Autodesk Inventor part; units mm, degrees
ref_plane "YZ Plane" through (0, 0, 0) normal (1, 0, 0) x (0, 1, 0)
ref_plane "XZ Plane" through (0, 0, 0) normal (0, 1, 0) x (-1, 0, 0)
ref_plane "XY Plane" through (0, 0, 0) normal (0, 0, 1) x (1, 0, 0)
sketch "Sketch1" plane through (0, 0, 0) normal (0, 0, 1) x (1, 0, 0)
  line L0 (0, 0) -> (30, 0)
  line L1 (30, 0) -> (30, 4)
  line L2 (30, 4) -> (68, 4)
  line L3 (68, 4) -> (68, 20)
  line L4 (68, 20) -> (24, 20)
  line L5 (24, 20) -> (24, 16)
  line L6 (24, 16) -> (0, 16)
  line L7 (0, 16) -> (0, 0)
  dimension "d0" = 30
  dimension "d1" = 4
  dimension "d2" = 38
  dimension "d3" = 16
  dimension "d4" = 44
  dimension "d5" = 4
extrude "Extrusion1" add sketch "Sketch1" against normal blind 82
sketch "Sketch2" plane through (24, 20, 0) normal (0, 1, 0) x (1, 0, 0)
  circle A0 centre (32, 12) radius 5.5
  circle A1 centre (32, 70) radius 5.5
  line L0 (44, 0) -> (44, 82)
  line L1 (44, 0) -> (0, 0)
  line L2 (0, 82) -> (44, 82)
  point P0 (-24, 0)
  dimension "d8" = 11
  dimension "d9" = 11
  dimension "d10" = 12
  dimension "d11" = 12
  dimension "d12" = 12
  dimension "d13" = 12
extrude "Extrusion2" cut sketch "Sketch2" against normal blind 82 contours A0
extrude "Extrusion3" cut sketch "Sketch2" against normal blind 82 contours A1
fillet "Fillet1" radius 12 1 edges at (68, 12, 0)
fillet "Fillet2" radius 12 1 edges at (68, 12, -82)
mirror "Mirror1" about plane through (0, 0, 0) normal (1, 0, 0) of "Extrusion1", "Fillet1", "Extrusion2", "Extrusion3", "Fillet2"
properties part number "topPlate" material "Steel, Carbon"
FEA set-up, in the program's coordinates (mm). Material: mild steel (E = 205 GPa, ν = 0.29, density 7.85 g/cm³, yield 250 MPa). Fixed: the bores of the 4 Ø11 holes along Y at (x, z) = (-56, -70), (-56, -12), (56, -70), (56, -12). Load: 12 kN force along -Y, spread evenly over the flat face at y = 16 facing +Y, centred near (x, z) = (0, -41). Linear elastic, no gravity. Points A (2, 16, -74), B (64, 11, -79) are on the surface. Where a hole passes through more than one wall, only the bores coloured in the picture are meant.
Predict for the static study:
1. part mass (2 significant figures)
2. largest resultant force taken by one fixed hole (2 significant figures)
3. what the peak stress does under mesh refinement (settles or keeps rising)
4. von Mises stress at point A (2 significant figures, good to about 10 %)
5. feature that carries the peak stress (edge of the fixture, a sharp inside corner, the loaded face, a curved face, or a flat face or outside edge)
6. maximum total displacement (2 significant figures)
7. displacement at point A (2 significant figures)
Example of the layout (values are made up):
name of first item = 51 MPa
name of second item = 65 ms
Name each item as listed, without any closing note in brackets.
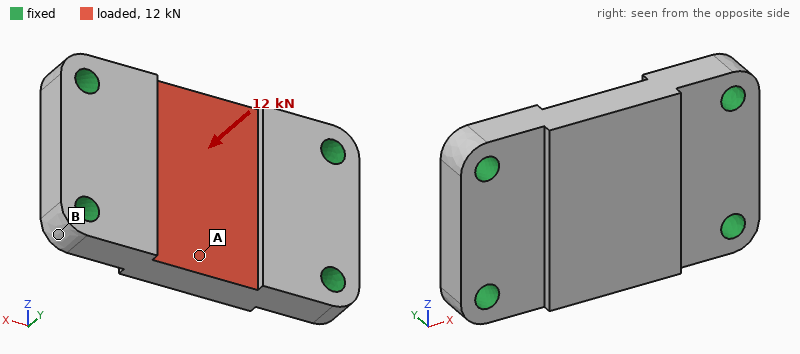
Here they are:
part mass = 1.4 kg
largest resultant force taken by one fixed hole = 4.0 kN
what the peak stress does under mesh refinement = keeps rising
von Mises stress at point A = 22 MPa
feature that carries the peak stress = edge of the fixture
maximum total displacement = 15 µm
displacement at point A = 15 µm
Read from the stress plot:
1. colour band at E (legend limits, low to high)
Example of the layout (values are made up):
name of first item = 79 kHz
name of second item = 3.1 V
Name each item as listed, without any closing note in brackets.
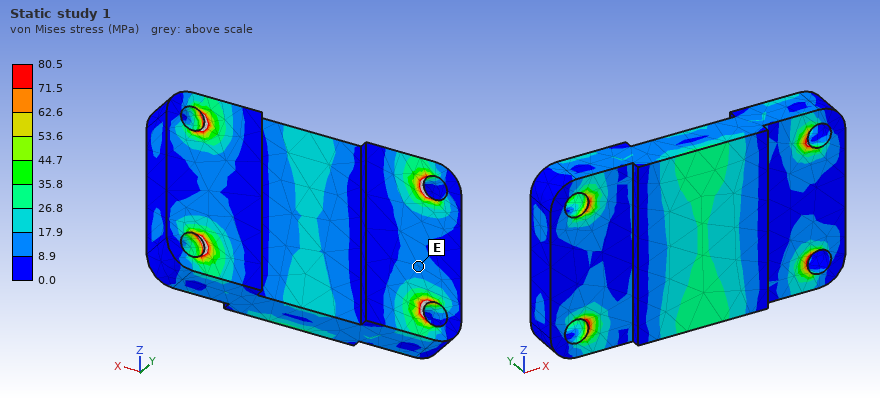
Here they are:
colour band at E = 8.9 to 17.9 MPa
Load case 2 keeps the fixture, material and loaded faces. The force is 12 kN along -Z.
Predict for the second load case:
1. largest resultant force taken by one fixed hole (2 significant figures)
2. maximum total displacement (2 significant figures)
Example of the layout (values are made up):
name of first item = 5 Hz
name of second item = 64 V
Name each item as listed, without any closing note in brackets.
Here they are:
largest resultant force taken by one fixed hole = 3.6 kN
maximum total displacement = 5.5 µm
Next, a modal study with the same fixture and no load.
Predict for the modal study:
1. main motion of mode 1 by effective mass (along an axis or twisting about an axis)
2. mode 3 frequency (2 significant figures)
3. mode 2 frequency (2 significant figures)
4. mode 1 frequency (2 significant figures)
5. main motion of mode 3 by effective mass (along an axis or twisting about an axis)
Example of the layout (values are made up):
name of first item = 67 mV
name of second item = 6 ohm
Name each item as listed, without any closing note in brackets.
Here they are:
main motion of mode 1 by effective mass = along Y
mode 3 frequency = 12 kHz
mode 2 frequency = 8200 Hz
mode 1 frequency = 6000 Hz
main motion of mode 3 by effective mass = along Z
